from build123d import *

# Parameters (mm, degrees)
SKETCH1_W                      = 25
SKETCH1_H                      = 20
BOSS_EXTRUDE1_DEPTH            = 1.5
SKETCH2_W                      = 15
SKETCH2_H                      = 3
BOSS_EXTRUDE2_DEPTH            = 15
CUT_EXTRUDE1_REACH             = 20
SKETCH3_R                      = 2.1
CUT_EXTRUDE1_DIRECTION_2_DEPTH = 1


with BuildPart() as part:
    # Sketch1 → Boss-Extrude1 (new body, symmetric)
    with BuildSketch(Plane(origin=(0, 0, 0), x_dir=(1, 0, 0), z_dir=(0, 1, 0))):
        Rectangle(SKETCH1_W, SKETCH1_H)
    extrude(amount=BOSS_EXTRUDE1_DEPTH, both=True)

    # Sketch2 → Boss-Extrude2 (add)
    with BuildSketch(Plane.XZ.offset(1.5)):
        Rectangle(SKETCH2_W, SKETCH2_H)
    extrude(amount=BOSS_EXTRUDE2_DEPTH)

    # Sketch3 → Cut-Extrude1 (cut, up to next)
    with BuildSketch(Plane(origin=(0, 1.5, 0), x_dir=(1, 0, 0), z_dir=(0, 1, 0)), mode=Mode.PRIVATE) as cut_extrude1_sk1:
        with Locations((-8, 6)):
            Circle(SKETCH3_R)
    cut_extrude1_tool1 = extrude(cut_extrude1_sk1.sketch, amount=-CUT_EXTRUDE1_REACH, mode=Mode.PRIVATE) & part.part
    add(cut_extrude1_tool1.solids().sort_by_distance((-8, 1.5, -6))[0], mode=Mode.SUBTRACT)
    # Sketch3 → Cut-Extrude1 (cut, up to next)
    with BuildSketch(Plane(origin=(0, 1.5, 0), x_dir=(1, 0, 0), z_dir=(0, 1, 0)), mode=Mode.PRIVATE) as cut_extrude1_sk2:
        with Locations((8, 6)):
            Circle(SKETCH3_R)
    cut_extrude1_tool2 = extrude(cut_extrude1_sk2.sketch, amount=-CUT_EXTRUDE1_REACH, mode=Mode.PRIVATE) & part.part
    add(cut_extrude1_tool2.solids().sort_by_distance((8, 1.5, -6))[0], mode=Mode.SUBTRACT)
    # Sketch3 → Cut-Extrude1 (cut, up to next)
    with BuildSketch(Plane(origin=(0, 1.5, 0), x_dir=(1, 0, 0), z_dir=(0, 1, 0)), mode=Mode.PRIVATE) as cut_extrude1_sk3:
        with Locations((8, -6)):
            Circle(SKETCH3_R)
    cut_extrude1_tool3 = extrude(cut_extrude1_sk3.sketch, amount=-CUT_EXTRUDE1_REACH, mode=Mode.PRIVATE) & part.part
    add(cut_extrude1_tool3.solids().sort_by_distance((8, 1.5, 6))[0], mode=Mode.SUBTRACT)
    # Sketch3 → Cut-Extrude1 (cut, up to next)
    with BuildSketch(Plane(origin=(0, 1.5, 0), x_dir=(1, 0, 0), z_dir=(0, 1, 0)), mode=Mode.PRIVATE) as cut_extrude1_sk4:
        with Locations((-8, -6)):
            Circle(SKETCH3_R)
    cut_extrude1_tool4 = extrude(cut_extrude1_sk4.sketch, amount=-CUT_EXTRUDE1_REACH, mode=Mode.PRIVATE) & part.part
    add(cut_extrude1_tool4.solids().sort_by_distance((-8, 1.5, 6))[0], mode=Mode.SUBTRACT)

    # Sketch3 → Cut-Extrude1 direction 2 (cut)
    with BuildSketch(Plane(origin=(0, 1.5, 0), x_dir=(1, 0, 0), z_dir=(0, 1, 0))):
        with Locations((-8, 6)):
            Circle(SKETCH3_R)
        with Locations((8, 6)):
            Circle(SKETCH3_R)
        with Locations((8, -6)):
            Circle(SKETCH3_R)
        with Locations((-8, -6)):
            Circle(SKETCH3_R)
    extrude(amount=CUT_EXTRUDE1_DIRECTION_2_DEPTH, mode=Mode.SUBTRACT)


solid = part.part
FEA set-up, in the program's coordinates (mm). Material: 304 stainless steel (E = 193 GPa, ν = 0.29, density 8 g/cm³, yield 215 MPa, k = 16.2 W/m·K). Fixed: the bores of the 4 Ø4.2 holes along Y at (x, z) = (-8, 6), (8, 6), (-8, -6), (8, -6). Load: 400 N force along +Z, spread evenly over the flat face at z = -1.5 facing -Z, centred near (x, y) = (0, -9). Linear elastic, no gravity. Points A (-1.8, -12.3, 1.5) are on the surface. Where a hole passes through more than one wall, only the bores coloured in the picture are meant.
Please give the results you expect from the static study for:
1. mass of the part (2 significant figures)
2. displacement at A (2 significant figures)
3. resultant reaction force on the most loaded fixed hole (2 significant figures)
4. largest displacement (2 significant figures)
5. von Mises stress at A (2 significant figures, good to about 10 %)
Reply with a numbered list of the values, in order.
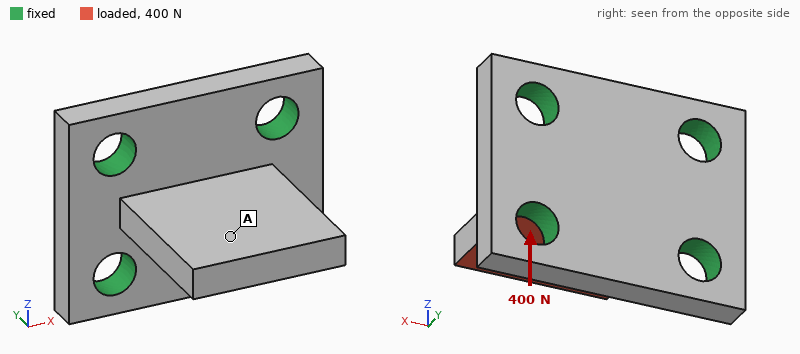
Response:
1. 16 g
2. 24 µm
3. 240 N
4. 36 µm
5. 12 MPa
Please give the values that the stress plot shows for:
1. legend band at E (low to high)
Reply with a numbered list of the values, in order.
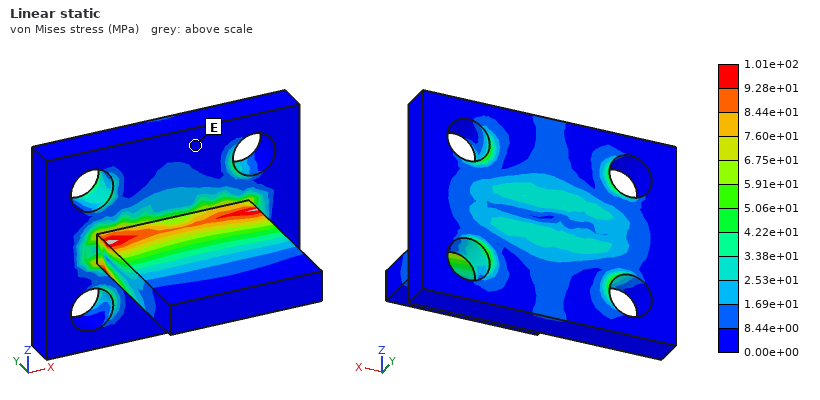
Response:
1. 0.00e+00 to 8.44e+00 MPa
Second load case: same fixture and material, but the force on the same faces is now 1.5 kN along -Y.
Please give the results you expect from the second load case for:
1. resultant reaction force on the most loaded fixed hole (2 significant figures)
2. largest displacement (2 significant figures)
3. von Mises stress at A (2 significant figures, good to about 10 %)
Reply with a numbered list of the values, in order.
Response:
1. 520 N
2. 33 µm
3. 19 MPa
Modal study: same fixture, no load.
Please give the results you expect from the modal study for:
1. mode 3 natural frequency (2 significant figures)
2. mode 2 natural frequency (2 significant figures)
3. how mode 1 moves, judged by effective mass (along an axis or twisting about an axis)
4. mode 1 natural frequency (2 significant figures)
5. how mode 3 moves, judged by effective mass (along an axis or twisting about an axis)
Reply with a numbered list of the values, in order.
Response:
1. 25 kHz
2. 22 kHz
3. along Z
4. 8900 Hz
5. along X
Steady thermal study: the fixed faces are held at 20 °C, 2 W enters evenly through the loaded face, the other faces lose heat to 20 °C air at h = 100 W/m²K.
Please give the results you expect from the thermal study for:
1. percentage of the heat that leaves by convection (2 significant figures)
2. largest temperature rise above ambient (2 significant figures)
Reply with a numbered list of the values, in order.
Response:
1. 32 %
2. 20 K
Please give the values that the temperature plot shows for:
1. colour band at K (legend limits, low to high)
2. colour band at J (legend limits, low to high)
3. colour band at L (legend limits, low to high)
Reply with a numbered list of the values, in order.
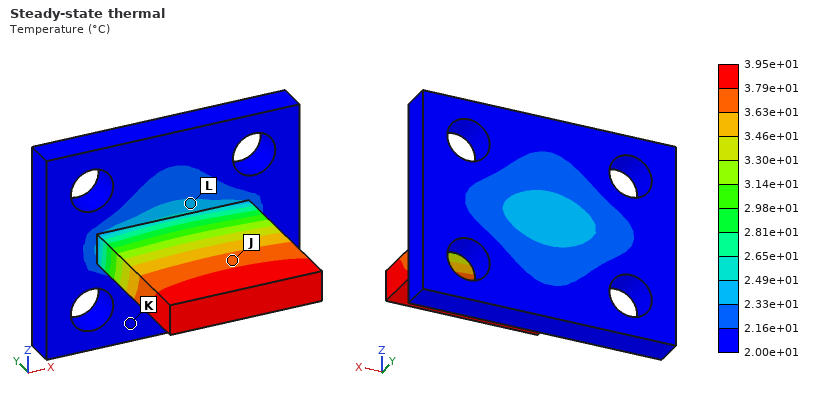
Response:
1. 2.00e+01 to 2.16e+01 °C
2. 3.63e+01 to 3.79e+01 °C
3. 2.33e+01 to 2.49e+01 °C
